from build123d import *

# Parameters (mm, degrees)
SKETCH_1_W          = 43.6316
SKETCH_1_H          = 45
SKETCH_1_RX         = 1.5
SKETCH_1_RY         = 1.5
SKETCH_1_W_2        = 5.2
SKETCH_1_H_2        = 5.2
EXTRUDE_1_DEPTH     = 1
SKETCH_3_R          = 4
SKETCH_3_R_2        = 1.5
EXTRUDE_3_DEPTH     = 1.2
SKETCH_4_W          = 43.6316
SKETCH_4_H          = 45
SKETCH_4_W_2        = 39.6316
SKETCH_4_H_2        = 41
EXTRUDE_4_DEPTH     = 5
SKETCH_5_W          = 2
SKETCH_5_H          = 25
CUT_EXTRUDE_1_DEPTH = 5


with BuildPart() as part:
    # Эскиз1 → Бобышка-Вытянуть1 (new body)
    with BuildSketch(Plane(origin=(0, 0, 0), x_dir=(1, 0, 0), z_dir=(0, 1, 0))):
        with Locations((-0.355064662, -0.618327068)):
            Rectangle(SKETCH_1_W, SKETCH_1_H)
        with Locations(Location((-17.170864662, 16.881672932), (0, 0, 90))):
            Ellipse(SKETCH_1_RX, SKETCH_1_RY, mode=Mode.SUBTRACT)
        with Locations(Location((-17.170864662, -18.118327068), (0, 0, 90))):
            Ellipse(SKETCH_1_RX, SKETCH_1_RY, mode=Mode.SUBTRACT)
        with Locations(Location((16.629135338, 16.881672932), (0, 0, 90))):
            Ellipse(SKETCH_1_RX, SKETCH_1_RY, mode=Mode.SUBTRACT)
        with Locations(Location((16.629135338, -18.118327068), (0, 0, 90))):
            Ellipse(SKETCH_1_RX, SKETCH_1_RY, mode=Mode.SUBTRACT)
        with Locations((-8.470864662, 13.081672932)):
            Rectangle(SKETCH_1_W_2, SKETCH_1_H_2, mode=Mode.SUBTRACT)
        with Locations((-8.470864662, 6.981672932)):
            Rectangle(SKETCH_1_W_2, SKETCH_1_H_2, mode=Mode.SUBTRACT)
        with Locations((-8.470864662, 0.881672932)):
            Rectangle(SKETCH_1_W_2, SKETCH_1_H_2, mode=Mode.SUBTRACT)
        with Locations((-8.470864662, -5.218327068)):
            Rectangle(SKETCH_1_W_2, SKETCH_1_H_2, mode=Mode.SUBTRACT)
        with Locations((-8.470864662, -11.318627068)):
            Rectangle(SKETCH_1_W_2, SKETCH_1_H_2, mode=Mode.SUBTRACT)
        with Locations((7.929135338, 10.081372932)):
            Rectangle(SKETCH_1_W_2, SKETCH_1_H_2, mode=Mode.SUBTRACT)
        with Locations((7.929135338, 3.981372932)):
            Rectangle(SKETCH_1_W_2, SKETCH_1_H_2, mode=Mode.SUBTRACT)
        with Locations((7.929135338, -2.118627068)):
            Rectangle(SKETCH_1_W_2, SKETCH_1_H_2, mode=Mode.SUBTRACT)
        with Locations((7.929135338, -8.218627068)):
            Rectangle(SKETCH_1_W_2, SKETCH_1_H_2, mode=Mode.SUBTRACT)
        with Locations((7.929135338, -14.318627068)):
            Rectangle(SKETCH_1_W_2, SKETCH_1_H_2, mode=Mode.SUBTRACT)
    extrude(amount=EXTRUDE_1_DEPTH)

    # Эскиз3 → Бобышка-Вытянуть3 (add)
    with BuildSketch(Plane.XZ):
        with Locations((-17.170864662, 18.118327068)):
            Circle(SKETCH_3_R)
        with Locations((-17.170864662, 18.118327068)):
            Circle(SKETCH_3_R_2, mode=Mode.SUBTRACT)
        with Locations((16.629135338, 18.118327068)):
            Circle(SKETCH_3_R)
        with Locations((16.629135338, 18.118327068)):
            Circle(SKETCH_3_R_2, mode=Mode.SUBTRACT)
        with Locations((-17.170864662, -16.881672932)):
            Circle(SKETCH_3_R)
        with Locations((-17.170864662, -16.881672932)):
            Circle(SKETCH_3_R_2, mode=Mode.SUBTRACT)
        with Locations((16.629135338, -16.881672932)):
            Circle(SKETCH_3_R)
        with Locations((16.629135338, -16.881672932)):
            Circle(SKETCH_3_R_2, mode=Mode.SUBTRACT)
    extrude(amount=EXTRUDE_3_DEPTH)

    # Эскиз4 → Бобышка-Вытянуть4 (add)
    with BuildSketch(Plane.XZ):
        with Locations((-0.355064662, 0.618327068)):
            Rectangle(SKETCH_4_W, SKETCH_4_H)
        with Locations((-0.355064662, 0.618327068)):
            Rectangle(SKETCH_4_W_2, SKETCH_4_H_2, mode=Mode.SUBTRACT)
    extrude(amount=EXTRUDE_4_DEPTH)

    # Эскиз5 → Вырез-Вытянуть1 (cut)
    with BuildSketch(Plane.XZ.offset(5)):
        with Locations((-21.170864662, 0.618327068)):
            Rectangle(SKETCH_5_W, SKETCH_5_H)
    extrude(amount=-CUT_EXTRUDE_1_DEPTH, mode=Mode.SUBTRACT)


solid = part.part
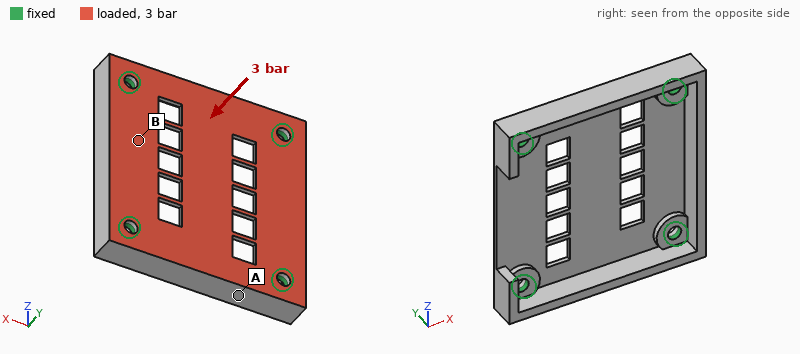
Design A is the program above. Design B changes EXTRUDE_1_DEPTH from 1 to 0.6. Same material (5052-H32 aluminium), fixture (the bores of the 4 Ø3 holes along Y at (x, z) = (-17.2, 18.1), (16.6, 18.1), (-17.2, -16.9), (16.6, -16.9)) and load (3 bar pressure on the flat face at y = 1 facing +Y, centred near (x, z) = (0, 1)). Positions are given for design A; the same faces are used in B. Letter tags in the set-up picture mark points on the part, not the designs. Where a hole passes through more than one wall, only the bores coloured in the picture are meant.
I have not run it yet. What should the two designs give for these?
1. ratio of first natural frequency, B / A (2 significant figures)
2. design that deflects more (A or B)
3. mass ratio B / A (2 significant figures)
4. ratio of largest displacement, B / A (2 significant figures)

0.65
B
0.80
3.9
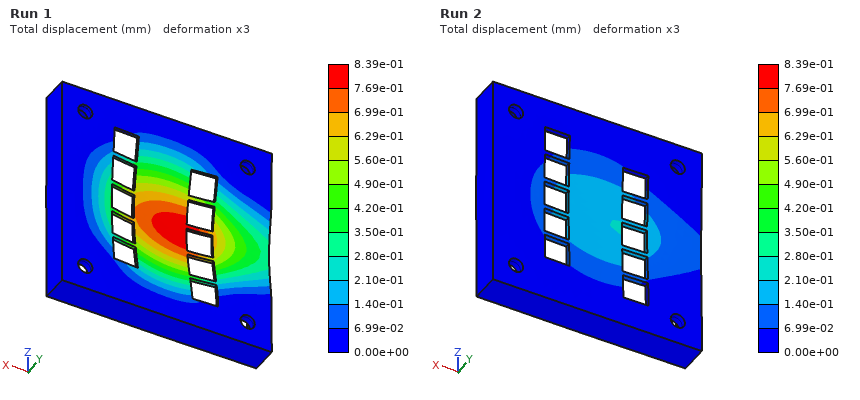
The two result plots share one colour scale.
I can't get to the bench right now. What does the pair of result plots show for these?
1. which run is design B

Run 1
